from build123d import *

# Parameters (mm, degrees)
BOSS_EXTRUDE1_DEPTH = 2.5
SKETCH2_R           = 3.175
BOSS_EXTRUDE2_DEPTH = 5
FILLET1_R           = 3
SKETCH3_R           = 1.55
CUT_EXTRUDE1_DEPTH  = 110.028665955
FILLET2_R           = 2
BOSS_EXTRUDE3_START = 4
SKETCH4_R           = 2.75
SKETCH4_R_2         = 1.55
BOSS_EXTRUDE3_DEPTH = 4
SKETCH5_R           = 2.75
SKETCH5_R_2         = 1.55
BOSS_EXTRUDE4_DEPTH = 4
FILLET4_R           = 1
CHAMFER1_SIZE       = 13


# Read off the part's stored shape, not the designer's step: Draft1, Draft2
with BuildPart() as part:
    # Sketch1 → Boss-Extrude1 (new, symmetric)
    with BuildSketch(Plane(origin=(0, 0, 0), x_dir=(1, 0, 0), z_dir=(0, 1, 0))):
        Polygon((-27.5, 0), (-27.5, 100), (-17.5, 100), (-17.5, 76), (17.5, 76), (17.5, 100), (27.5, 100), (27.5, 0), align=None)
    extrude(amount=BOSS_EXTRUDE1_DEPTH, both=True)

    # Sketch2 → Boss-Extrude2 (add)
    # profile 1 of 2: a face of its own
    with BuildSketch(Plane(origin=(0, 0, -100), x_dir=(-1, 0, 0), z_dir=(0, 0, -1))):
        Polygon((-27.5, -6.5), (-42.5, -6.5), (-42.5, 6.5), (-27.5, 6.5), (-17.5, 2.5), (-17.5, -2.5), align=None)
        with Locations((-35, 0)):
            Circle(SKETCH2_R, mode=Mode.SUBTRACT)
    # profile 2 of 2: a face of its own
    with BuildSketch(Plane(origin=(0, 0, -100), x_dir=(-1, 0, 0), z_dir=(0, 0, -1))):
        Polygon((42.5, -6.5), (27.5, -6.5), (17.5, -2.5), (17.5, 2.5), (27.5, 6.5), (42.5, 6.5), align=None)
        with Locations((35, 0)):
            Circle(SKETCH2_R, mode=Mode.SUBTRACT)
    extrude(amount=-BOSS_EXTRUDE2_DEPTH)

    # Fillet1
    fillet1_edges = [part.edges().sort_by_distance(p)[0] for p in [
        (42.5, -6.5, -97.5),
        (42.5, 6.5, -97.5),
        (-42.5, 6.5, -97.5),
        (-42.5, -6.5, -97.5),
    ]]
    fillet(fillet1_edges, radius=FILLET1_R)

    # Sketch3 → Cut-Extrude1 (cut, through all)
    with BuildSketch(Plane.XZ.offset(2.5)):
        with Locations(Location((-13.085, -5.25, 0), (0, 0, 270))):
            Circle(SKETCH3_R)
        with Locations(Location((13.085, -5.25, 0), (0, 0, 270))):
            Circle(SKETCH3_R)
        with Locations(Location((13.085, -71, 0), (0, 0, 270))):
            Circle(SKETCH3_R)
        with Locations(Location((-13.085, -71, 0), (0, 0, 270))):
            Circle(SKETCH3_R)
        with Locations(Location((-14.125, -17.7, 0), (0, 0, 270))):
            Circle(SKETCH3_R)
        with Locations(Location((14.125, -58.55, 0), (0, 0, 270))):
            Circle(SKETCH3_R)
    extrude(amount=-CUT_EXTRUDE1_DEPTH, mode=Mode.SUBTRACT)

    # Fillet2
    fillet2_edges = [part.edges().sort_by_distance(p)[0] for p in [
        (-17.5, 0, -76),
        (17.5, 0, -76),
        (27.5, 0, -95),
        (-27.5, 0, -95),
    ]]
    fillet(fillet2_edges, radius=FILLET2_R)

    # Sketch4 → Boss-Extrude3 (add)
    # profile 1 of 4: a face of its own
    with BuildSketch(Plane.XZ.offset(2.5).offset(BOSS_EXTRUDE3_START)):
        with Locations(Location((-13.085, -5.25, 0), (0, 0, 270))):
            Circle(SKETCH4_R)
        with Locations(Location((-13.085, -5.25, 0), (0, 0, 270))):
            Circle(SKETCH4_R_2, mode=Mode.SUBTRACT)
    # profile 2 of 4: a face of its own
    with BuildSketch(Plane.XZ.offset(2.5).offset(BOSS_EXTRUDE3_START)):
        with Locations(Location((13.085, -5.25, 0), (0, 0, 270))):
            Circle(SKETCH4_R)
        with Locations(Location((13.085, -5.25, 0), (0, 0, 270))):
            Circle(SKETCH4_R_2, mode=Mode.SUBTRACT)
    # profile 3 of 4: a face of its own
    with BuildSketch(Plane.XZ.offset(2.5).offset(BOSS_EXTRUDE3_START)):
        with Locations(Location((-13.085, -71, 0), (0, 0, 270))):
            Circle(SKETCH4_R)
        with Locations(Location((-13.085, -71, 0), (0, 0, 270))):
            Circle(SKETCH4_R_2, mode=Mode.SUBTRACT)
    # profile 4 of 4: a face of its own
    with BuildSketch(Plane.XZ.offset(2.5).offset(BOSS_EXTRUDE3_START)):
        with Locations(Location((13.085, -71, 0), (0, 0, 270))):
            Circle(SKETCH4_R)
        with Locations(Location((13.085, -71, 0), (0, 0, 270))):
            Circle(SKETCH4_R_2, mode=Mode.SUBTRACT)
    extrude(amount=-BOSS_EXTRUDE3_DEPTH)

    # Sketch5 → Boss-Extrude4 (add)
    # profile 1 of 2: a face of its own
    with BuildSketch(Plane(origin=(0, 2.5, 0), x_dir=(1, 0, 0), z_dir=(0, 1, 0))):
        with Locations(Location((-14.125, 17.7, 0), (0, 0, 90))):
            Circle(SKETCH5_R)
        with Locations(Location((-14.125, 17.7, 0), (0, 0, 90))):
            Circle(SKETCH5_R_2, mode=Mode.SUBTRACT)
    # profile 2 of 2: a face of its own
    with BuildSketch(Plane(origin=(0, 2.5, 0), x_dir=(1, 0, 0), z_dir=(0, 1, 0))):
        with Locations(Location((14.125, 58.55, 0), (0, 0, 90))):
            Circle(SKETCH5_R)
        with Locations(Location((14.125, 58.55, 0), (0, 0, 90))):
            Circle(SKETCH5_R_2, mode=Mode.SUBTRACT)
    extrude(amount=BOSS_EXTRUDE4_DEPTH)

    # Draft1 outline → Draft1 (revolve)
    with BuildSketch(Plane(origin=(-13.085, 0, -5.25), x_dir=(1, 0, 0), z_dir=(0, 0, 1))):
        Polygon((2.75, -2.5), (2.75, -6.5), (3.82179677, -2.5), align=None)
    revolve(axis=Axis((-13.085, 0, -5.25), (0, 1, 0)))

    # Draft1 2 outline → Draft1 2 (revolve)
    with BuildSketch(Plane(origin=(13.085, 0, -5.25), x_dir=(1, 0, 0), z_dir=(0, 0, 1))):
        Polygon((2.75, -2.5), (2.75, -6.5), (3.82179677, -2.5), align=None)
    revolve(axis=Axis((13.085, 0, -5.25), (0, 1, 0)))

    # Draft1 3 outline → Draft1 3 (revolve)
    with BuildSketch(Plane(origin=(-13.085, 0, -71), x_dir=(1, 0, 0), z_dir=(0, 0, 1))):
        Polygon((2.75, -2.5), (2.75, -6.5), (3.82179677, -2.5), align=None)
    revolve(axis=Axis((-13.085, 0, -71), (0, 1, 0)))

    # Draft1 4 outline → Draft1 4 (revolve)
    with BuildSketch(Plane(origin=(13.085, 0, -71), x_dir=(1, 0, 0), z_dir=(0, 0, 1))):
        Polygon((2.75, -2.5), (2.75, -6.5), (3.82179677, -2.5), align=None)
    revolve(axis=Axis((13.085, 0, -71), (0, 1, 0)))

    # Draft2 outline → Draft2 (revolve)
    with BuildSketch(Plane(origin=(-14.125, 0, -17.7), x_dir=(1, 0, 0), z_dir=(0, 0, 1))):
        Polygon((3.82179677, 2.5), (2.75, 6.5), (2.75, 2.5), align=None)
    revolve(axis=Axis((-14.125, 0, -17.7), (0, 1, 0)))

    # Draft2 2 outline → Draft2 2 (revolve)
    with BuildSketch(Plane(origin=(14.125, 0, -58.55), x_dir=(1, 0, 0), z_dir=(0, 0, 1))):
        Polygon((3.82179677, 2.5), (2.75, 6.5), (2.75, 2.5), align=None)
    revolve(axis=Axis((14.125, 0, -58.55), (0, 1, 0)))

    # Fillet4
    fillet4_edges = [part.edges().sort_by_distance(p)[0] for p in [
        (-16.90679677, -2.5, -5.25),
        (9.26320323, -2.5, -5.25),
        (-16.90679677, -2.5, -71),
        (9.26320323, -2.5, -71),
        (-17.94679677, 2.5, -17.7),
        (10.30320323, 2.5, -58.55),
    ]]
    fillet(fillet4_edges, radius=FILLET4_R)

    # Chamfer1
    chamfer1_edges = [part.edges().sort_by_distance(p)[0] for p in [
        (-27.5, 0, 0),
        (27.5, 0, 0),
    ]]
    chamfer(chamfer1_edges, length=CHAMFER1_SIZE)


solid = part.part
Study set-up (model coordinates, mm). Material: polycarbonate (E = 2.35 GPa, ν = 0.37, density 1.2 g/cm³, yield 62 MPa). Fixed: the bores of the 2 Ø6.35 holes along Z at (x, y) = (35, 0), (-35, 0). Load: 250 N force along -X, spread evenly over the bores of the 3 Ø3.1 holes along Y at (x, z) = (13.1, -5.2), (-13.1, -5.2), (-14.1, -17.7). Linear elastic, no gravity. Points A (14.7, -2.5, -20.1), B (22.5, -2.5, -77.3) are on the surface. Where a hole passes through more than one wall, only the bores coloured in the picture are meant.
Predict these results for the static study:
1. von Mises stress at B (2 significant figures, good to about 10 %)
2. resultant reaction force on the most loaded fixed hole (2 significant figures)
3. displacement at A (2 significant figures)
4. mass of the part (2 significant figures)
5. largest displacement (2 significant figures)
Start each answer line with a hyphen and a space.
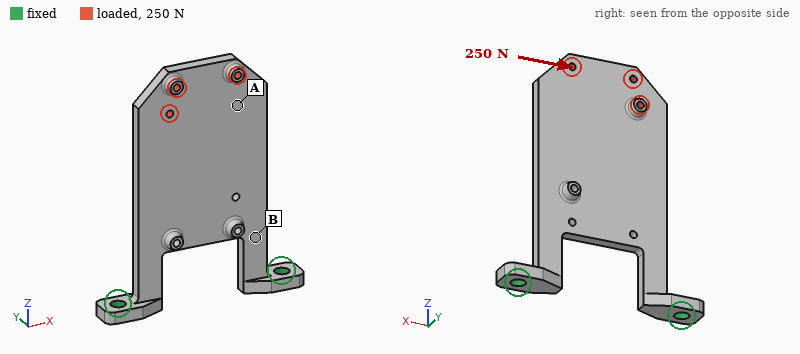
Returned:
- 8.1 MPa
- 410 N
- 0.87 mm
- 30 g
- 1.1 mm
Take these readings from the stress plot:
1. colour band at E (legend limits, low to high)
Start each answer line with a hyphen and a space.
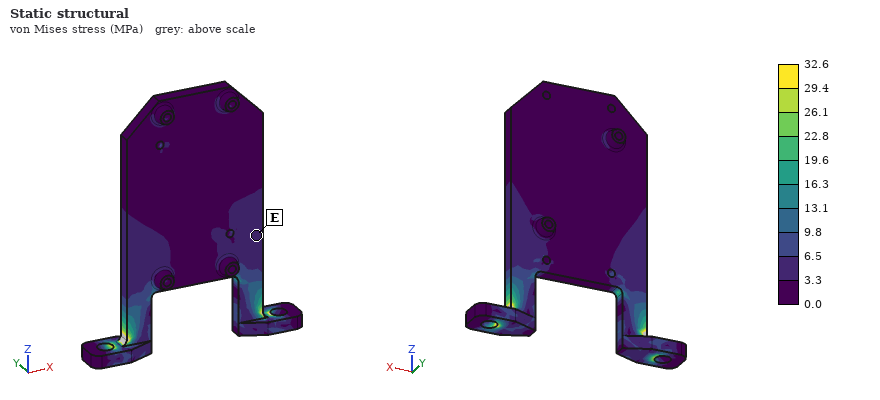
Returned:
- 3.3 to 6.5 MPa
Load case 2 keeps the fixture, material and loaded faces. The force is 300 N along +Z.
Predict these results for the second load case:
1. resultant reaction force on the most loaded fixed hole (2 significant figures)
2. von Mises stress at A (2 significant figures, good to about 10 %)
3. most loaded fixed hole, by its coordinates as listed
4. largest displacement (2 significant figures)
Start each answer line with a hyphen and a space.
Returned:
- 180 N
- 2.2 MPa
- (-35, 0)
- 1.5 mm
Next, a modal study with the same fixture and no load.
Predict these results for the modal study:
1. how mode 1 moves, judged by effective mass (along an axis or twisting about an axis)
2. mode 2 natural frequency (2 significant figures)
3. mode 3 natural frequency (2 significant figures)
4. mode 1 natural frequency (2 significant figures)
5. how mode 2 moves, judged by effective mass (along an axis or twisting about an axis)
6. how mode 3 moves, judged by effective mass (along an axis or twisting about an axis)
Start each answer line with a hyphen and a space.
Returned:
- along Y
- 410 Hz
- 620 Hz
- 76 Hz
- twisting about Z
- along Y
